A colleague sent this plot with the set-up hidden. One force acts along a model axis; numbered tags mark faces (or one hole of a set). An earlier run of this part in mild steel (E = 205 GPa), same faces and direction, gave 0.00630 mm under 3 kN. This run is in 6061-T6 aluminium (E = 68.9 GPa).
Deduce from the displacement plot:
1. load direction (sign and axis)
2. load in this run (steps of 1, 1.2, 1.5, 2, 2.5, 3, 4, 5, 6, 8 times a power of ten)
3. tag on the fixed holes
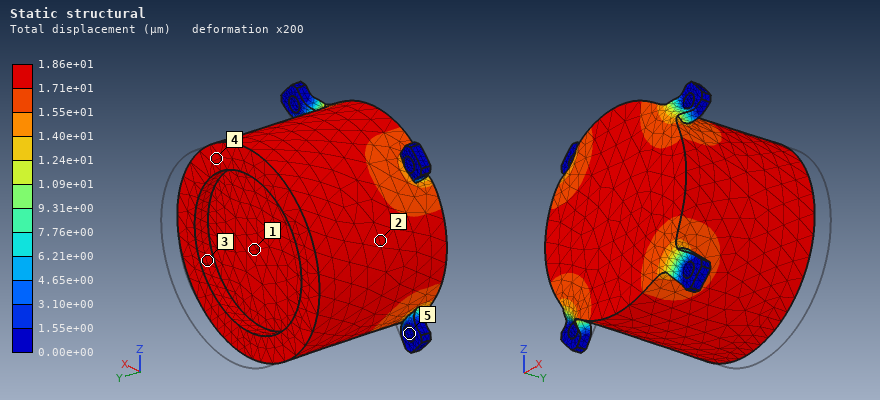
-Y
3 kN
5
